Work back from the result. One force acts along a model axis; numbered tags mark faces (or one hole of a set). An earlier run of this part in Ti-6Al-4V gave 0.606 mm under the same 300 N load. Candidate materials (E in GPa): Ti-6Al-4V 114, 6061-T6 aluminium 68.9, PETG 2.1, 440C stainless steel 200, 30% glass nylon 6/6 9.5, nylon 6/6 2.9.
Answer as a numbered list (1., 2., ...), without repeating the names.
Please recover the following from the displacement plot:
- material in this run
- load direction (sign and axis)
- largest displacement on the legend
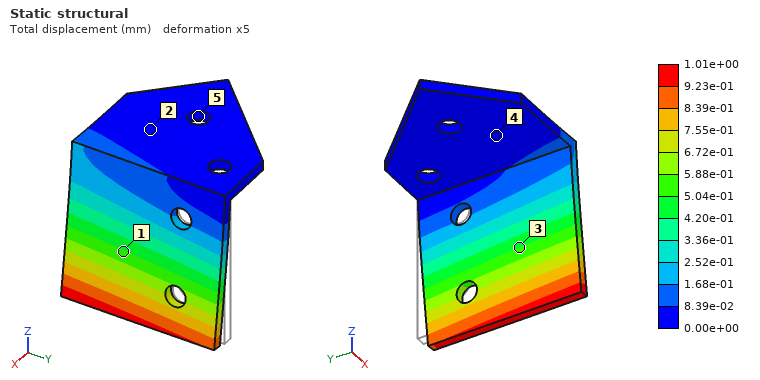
1. 6061-T6 aluminium
2. +X
3. 1.01e+00 mm
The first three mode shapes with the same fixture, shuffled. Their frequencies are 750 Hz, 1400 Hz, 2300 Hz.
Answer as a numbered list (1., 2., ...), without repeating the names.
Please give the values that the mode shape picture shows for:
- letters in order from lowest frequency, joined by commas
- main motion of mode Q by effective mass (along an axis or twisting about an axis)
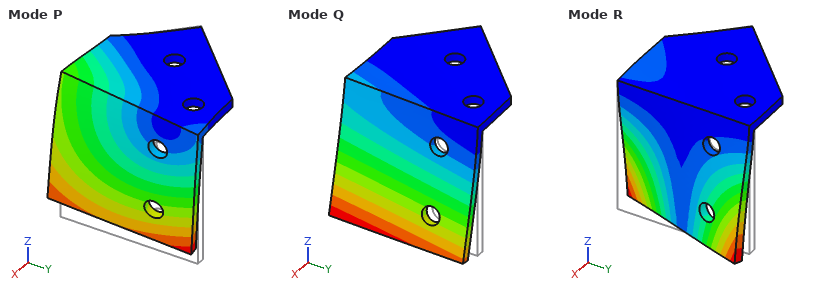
1. Q, P, R
2. along X
